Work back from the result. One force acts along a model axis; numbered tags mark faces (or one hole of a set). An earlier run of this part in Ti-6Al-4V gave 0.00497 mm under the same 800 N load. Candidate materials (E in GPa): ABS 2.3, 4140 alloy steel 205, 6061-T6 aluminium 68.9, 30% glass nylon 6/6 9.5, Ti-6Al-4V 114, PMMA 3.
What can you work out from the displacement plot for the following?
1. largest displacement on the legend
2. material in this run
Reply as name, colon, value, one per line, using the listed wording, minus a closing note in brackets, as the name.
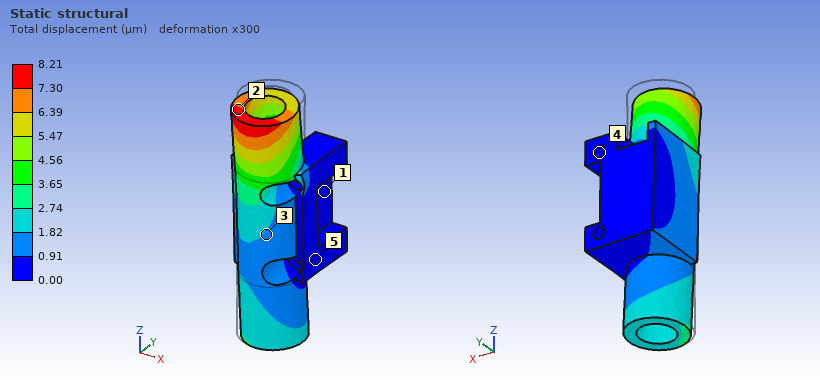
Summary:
largest displacement on the legend: 8.21 µm
material in this run: 6061-T6 aluminium
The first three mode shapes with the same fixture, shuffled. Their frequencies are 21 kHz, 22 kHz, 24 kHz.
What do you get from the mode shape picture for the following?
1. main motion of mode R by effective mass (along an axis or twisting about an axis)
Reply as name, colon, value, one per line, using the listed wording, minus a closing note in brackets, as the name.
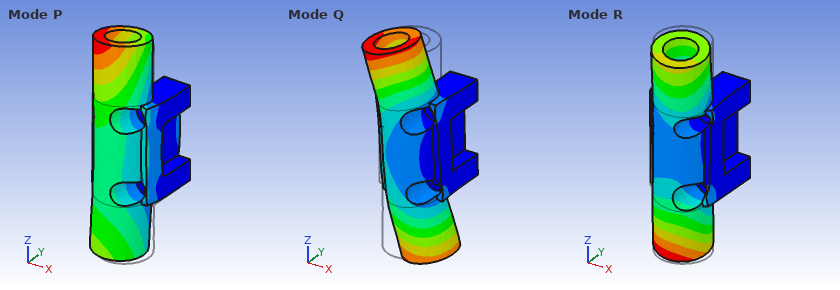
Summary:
main motion of mode R by effective mass: twisting about X
